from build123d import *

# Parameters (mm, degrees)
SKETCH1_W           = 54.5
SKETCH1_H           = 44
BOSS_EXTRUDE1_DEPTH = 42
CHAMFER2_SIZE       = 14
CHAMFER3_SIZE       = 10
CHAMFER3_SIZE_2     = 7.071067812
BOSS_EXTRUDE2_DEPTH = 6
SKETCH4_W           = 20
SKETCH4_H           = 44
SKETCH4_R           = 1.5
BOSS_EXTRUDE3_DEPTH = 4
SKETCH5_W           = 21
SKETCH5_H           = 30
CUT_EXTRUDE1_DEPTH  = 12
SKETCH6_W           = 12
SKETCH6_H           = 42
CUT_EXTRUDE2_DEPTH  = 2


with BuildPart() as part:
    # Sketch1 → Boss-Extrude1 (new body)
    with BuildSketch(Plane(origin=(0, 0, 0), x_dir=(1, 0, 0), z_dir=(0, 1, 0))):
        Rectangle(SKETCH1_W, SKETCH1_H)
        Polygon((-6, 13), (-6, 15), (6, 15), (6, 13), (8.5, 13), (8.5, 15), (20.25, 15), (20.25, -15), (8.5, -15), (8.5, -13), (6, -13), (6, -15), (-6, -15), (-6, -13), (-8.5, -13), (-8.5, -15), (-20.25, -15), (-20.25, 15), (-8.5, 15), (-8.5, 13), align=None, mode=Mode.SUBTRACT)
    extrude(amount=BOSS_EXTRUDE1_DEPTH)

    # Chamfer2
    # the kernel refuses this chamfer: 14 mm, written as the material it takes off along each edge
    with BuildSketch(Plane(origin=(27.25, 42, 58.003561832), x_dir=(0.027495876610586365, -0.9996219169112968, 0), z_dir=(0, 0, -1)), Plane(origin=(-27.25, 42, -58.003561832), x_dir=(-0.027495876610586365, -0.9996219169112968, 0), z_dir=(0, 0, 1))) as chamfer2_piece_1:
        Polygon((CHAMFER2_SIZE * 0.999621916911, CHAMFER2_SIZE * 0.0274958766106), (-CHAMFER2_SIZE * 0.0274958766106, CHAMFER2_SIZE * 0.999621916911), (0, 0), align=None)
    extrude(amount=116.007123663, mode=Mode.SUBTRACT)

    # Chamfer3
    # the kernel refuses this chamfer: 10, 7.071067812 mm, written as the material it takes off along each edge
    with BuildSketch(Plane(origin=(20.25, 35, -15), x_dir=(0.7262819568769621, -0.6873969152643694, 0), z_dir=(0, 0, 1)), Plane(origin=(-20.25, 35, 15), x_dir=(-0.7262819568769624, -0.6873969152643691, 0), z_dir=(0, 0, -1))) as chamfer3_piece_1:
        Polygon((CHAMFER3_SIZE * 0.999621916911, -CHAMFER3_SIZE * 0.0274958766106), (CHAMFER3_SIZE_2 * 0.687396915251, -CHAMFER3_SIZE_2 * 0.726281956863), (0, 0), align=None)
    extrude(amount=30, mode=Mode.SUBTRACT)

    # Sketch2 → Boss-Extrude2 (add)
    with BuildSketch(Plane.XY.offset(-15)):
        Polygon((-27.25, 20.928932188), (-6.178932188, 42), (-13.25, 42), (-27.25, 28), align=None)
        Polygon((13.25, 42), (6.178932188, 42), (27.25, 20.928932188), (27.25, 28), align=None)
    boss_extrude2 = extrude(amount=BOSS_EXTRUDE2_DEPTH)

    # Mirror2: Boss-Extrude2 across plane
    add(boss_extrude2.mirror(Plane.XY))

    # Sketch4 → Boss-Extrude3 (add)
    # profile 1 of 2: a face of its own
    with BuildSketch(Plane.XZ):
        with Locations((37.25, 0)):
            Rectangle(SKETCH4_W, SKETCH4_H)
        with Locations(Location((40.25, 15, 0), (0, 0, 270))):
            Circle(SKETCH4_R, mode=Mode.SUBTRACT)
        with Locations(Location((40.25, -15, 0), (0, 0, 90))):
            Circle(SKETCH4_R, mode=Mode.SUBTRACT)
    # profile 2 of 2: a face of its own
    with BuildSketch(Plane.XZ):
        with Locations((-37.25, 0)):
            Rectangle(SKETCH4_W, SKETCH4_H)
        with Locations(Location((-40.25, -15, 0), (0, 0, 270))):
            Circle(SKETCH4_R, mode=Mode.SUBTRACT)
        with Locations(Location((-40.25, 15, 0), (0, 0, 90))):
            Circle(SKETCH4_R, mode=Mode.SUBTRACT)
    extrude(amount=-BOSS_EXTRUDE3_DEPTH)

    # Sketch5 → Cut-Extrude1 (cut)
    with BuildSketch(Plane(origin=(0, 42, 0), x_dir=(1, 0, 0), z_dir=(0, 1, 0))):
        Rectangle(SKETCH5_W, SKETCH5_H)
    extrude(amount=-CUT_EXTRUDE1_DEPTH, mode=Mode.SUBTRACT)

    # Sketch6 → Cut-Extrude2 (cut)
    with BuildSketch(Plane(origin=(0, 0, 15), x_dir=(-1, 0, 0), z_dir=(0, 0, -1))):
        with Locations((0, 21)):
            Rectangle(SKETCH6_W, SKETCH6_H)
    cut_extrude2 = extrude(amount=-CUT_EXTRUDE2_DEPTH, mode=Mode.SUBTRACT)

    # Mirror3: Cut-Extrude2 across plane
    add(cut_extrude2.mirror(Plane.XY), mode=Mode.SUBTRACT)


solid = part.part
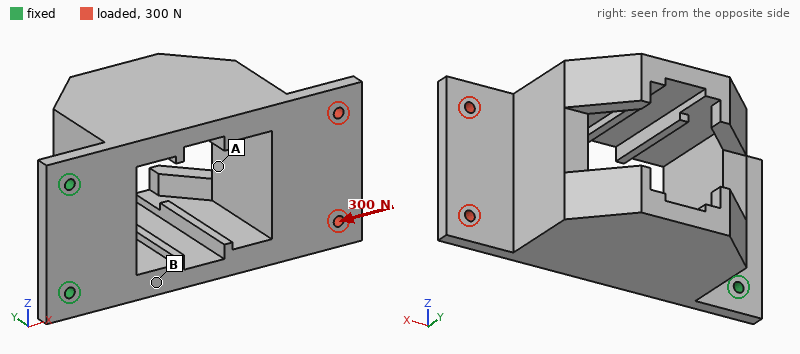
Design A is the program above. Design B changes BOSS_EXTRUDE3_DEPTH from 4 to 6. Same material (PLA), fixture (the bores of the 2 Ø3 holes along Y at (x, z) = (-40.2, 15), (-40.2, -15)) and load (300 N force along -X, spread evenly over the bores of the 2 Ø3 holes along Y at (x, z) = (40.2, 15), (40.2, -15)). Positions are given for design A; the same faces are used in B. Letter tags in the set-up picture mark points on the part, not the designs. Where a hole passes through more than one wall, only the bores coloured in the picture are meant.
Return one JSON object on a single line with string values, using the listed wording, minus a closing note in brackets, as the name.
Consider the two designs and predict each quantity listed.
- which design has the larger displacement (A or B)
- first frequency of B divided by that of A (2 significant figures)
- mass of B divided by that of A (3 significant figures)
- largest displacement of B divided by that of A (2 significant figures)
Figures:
{"which design has the larger displacement": "A", "first frequency of B divided by that of A": "1.6", "mass of B divided by that of A": "1.07", "largest displacement of B divided by that of A": "0.74"}
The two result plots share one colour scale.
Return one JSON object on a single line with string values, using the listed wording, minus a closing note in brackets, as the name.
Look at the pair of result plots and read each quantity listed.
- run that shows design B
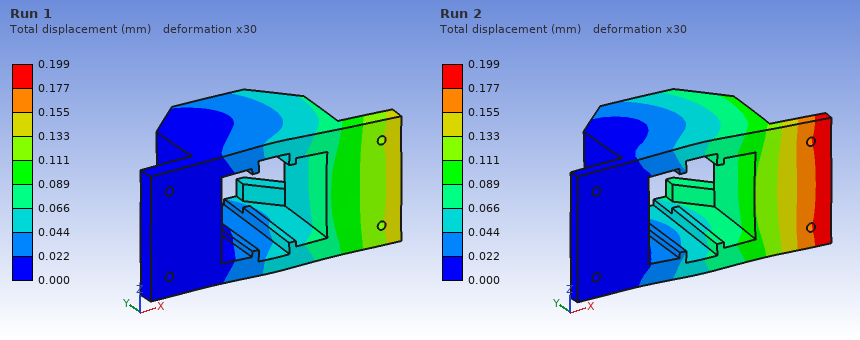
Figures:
{"run that shows design B": "Run 1"}
